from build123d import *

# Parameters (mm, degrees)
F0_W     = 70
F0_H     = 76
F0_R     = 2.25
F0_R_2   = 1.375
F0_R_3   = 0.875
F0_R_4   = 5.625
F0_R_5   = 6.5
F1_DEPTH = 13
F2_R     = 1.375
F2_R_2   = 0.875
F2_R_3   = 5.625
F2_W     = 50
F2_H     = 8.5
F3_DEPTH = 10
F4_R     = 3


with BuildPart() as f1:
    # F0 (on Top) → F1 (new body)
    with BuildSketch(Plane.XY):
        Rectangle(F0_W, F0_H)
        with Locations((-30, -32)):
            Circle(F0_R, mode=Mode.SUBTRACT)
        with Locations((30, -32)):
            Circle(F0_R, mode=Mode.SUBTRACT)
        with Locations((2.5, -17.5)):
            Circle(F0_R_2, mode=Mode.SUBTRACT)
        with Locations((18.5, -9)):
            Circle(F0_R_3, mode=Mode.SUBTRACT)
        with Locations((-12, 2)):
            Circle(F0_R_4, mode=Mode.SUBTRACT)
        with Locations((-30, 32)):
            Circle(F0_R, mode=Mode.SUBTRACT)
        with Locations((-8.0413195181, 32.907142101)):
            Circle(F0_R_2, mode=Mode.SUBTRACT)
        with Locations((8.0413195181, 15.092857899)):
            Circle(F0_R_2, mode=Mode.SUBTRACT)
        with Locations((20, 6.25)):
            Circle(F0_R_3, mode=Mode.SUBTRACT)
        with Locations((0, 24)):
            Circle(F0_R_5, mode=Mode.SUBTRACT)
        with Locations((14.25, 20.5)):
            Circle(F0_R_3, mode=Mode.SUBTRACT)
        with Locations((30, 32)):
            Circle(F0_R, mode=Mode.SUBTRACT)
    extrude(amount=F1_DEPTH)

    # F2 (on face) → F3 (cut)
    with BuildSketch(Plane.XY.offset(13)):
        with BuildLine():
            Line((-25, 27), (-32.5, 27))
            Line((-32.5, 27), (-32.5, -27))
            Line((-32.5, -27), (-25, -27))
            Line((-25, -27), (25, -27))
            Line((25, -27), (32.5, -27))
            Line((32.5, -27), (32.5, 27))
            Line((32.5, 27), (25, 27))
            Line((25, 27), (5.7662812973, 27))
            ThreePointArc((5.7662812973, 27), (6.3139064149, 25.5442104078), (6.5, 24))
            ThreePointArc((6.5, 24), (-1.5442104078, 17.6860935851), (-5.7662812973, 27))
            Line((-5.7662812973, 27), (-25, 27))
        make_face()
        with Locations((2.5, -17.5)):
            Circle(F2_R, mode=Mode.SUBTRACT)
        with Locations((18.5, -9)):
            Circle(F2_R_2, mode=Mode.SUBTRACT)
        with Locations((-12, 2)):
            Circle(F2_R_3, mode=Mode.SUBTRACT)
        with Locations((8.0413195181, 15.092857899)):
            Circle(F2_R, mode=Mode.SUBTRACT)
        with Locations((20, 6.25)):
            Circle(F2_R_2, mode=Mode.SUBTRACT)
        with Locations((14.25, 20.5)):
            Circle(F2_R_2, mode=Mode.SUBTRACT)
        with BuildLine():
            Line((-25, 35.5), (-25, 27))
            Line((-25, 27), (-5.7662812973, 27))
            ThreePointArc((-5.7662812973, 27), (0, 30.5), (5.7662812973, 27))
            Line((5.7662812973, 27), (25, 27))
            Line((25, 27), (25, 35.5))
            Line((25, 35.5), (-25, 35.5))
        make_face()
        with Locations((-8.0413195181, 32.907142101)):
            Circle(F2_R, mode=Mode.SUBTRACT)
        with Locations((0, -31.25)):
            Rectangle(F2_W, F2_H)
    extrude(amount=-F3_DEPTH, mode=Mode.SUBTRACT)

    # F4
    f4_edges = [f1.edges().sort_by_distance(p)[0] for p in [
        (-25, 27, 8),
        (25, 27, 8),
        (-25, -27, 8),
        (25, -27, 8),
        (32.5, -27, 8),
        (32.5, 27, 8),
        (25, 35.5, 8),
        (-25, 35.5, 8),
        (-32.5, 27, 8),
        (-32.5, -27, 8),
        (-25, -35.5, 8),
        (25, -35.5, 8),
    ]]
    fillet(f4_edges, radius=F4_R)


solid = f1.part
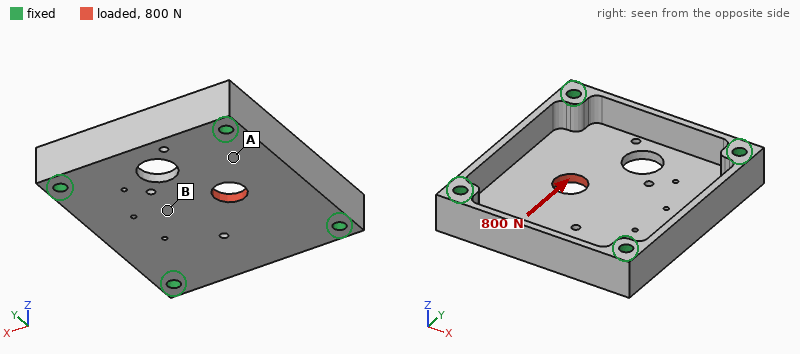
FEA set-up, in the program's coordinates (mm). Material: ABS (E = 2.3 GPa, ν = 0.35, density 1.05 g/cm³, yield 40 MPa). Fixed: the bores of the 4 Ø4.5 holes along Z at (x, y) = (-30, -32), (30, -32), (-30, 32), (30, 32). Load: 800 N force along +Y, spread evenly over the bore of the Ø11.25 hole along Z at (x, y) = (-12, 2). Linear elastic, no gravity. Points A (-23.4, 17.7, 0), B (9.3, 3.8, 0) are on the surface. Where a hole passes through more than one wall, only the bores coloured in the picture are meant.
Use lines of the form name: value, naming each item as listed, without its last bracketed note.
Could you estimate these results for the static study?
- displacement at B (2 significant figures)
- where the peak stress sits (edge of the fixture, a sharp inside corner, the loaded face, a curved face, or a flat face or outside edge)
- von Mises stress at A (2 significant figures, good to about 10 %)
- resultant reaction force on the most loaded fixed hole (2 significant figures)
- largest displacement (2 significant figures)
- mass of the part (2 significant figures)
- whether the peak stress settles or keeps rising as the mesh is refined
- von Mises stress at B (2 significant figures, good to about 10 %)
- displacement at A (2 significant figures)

displacement at B: 36 µm
where the peak stress sits: edge of the fixture
von Mises stress at A: 4.9 MPa
resultant reaction force on the most loaded fixed hole: 300 N
largest displacement: 99 µm
mass of the part: 25 g
whether the peak stress settles or keeps rising as the mesh is refined: keeps rising
von Mises stress at B: 1.6 MPa
displacement at A: 37 µm
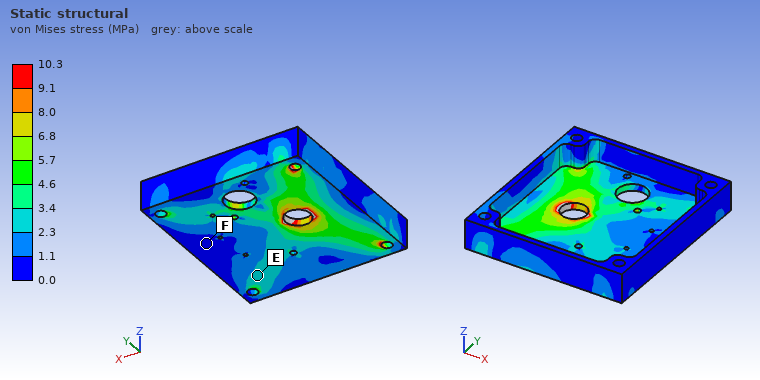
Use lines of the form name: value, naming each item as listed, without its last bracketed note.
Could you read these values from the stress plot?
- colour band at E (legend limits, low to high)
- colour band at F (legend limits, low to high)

colour band at E: 2.3 to 3.4 MPa
colour band at F: 0.0 to 1.1 MPa
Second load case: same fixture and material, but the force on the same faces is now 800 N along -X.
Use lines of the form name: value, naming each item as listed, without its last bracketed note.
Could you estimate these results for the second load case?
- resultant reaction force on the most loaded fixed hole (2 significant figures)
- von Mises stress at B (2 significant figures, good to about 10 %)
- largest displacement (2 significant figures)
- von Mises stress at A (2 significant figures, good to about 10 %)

resultant reaction force on the most loaded fixed hole: 240 N
von Mises stress at B: 2.6 MPa
largest displacement: 0.14 mm
von Mises stress at A: 4.8 MPa
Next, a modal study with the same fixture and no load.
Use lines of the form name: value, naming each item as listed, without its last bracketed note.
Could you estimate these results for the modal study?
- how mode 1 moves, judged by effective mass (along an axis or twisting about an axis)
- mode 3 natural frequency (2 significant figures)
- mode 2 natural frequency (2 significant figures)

how mode 1 moves, judged by effective mass: along Z
mode 3 natural frequency: 2300 Hz
mode 2 natural frequency: 2300 Hz
